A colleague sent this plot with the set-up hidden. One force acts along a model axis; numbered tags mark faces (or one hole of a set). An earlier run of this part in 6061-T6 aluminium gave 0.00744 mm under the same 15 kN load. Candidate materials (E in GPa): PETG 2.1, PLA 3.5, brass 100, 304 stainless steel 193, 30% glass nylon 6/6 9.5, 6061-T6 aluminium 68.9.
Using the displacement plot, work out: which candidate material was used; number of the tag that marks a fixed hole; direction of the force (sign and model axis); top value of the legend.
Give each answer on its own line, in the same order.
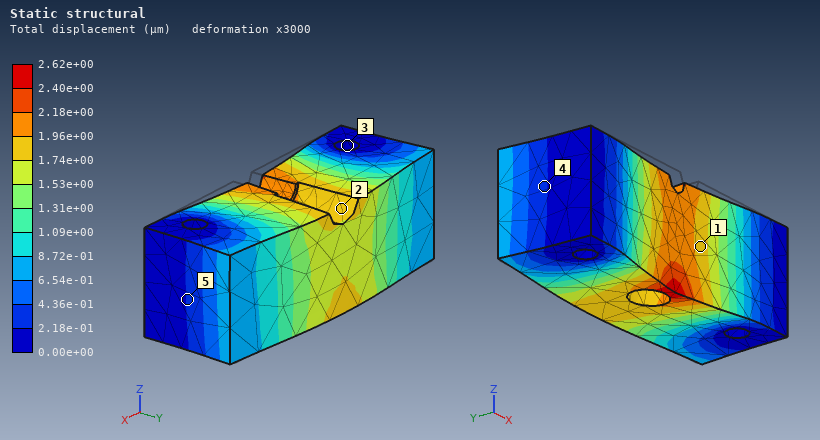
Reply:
304 stainless steel
3
+Y
2.62e+00 µm
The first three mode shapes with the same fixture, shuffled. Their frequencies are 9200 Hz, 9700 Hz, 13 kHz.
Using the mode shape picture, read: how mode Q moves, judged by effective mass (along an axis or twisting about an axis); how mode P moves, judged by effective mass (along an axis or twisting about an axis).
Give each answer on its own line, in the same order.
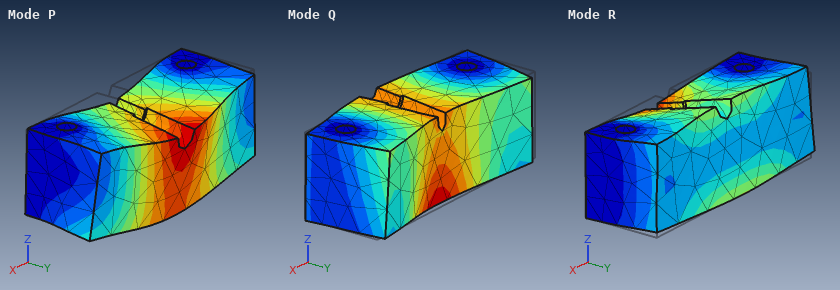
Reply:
along Y
along Z
